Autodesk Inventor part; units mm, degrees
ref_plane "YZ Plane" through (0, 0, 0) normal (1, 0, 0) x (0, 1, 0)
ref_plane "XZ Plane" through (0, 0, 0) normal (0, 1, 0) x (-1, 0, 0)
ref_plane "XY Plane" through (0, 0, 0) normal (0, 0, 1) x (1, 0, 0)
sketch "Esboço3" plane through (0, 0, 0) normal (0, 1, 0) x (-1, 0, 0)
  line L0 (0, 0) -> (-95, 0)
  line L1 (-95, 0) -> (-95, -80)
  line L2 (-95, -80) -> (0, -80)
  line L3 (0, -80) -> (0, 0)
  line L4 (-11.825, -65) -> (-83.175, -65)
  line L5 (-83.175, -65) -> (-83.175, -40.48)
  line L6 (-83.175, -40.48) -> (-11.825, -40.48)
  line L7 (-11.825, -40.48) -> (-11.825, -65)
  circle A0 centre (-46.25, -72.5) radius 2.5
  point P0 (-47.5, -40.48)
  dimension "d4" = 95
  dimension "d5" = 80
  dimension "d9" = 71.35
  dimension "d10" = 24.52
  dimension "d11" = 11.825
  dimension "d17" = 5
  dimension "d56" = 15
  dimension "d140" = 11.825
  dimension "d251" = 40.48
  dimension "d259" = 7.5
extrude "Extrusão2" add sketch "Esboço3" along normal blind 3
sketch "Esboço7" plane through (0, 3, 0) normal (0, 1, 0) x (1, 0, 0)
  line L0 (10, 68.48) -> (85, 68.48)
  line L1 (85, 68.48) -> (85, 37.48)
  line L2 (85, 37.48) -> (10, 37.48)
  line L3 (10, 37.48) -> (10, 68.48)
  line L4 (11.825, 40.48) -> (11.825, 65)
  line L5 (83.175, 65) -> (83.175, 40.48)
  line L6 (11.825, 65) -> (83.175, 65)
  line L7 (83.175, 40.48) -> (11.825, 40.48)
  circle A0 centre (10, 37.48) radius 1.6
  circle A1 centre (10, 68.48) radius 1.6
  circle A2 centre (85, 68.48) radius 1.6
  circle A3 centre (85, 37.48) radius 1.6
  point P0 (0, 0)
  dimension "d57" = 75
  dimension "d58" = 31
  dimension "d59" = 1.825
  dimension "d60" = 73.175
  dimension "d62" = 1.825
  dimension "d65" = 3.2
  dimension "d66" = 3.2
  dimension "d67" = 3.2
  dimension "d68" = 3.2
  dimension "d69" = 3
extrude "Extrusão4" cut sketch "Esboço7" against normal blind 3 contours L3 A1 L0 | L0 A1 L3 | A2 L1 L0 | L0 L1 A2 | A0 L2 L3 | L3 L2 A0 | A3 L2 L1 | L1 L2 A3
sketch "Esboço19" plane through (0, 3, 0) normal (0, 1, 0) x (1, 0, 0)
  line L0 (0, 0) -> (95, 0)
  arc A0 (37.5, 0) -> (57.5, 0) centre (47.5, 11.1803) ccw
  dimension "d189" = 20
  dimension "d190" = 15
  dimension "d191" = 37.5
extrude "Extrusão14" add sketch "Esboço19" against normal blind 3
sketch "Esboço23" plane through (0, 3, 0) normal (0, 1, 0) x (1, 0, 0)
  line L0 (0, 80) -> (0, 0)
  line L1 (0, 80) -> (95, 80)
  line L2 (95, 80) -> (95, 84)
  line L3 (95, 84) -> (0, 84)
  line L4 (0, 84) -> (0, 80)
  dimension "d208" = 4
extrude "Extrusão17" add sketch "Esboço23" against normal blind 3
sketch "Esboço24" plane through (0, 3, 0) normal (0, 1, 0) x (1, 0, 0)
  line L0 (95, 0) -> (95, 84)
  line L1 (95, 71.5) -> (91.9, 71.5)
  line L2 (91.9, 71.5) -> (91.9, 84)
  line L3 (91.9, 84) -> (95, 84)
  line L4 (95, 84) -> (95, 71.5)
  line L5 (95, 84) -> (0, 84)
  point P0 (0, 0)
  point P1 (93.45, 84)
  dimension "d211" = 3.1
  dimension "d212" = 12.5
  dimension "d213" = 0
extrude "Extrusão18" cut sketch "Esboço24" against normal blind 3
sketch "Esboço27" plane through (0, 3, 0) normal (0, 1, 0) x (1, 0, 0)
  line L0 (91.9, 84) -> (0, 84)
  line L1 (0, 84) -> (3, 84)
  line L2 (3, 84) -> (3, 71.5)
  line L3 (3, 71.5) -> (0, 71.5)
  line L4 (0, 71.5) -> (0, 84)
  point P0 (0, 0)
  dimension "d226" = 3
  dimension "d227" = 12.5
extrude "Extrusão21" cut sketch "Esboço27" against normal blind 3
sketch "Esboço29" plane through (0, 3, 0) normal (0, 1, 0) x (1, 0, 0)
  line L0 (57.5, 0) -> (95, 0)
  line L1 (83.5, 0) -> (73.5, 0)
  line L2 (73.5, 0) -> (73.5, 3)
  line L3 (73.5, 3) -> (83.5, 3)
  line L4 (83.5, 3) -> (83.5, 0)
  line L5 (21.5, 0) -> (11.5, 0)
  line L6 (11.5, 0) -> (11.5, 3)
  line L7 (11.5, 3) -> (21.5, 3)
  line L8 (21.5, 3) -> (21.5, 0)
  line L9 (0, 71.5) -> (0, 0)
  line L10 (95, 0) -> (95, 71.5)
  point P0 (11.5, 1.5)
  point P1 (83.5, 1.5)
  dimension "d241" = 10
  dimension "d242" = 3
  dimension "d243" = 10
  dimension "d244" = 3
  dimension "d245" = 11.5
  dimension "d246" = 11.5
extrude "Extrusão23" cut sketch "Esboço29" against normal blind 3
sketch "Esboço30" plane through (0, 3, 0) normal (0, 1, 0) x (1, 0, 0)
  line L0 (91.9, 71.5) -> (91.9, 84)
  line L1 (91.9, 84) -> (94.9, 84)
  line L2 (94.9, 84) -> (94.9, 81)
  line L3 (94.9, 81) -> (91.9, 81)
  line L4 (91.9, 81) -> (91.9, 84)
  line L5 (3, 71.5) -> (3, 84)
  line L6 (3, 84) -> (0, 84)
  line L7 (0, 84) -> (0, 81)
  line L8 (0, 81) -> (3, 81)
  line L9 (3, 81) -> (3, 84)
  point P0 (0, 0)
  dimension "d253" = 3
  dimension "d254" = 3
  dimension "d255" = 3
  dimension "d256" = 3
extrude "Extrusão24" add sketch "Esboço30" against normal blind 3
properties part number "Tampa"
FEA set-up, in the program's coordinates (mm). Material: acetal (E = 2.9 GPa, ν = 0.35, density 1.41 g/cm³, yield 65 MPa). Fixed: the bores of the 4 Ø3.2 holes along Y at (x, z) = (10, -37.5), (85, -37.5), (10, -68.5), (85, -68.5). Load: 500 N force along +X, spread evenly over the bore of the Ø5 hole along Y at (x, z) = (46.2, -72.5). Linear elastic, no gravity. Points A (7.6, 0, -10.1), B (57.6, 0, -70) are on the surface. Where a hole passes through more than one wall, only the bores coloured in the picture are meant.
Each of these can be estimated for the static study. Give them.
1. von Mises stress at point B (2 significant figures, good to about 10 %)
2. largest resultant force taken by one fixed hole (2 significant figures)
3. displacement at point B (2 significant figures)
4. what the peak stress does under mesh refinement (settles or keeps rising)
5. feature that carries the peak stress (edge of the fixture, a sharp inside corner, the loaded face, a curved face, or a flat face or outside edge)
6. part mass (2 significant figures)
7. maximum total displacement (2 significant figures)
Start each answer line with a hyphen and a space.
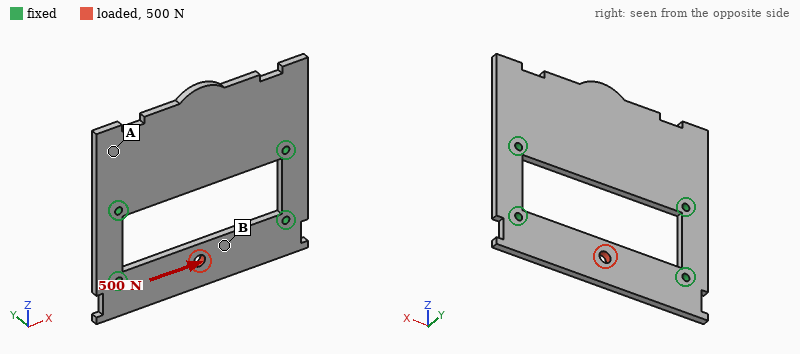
- 6.7 MPa
- 260 N
- 70 µm
- keeps rising
- edge of the fixture
- 26 g
- 95 µm
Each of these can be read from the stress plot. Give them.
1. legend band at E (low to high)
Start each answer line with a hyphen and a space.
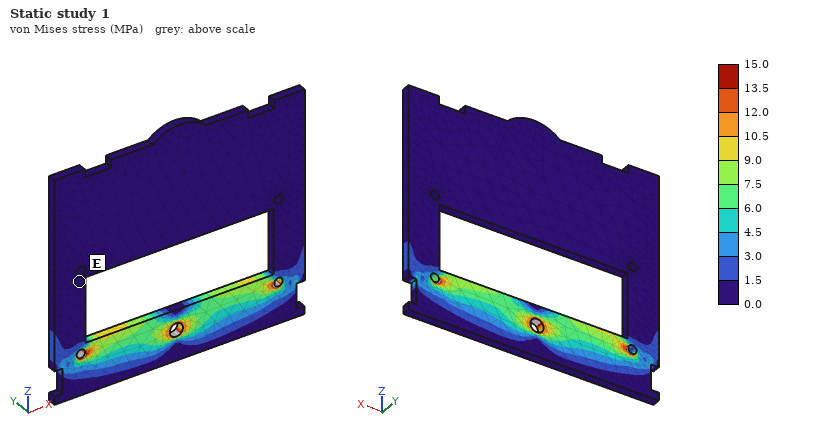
- 0.0 to 1.5 MPa
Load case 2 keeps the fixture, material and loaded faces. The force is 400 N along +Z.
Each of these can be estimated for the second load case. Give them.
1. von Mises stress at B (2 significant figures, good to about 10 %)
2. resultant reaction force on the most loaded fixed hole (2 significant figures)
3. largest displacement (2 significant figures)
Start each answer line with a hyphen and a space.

- 7.0 MPa
- 310 N
- 0.47 mm
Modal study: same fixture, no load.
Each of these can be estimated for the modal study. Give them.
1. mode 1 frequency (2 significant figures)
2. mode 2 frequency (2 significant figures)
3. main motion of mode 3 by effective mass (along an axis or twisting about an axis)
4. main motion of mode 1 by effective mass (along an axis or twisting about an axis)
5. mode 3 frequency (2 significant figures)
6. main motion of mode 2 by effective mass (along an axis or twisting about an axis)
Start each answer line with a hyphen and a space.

- 310 Hz
- 650 Hz
- along Y
- along Y
- 700 Hz
- twisting about Z
